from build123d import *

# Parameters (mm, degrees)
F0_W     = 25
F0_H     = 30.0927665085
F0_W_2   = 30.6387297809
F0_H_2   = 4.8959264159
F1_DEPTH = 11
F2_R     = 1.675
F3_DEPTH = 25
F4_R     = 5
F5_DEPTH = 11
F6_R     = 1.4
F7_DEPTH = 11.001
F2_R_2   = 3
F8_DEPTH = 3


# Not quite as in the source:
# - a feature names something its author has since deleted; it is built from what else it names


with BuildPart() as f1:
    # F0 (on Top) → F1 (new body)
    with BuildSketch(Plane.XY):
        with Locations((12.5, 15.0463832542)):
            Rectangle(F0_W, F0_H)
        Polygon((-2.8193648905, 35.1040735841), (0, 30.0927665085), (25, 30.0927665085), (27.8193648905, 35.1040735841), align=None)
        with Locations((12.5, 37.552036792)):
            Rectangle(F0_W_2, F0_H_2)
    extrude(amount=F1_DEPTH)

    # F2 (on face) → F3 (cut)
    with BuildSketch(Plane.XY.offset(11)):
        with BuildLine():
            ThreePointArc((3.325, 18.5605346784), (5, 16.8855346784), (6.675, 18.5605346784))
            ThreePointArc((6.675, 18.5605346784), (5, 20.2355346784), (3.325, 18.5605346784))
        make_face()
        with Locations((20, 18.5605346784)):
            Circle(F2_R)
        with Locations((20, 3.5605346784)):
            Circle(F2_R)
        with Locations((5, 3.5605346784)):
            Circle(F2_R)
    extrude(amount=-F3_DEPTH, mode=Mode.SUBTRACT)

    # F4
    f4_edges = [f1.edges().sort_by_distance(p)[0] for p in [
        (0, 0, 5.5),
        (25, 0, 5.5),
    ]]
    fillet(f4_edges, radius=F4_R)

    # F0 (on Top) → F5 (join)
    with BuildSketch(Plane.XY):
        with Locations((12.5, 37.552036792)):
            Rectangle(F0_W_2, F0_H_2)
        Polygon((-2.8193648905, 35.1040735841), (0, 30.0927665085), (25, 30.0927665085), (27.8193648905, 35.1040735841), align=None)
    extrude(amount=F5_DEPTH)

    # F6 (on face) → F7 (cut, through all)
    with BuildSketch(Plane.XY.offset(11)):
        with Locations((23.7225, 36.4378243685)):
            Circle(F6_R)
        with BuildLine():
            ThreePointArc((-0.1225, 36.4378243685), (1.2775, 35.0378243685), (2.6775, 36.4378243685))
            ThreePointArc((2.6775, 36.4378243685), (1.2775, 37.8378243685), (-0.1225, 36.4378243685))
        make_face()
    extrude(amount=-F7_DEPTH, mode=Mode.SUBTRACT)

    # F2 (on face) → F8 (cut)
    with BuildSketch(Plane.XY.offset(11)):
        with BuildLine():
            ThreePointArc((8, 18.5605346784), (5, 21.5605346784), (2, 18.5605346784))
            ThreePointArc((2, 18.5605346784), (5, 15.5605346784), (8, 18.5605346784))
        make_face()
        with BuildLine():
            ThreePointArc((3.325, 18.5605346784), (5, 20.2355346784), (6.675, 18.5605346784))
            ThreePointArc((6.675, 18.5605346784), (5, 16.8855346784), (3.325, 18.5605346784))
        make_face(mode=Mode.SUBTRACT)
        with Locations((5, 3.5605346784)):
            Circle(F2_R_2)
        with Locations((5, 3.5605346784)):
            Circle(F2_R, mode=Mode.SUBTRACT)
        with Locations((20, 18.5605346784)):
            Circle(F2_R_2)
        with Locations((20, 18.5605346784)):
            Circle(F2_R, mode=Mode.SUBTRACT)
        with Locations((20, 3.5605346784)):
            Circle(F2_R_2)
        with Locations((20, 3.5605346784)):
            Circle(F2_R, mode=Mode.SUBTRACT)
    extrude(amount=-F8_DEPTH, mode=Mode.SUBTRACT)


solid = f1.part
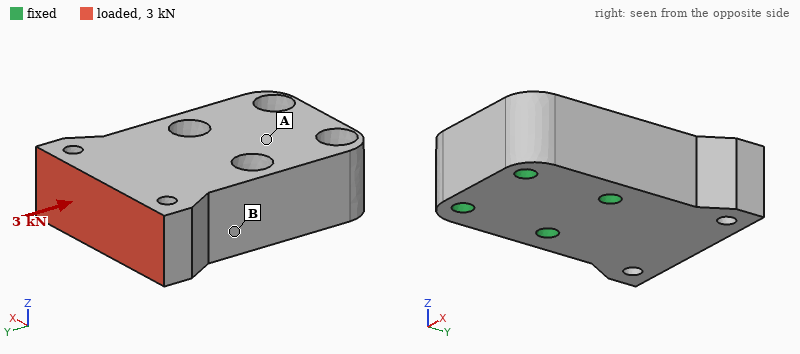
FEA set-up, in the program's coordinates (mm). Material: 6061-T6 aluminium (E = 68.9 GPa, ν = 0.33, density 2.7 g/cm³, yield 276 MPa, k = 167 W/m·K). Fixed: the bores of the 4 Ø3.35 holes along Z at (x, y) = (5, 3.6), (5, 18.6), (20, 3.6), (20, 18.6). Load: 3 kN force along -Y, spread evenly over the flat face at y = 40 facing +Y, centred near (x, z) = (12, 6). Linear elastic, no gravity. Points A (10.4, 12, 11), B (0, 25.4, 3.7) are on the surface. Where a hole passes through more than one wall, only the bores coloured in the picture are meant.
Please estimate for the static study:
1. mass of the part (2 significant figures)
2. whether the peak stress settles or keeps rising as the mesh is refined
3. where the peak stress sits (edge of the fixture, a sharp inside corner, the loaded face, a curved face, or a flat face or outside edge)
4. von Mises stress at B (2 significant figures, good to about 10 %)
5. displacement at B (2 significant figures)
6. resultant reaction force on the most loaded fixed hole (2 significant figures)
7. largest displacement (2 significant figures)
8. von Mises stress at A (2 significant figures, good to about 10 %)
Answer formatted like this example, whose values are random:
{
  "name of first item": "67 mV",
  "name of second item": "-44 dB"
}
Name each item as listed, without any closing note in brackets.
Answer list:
{
  "mass of the part": "29 g",
  "whether the peak stress settles or keeps rising as the mesh is refined": "keeps rising",
  "where the peak stress sits": "edge of the fixture",
  "von Mises stress at B": "13 MPa",
  "displacement at B": "1.6 µm",
  "resultant reaction force on the most loaded fixed hole": "1.3 kN",
  "largest displacement": "6.6 µm",
  "von Mises stress at A": "5.1 MPa"
}
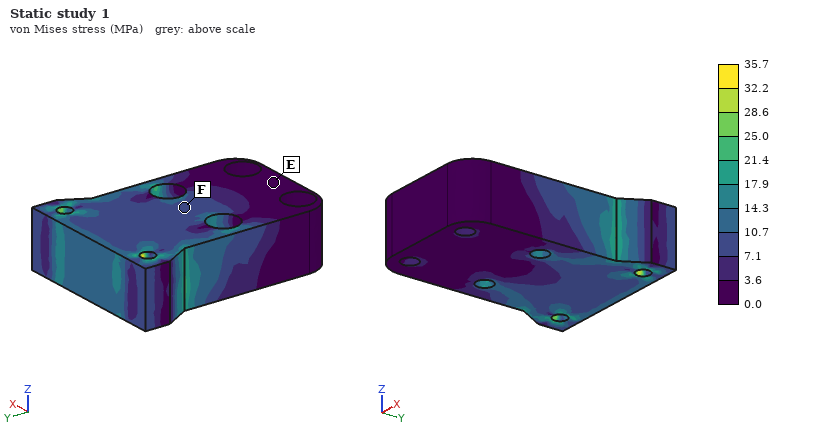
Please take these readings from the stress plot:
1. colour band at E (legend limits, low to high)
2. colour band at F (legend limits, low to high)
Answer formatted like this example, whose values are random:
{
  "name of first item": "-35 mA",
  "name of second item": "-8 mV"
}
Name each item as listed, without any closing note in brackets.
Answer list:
{
  "colour band at E": "0.0 to 3.6 MPa",
  "colour band at F": "7.1 to 10.7 MPa"
}
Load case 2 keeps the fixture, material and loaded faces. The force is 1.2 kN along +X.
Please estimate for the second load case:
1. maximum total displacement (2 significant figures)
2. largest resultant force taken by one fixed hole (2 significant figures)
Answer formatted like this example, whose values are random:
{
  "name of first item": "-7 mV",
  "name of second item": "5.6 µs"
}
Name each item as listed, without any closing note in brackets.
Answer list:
{
  "maximum total displacement": "12 µm",
  "largest resultant force taken by one fixed hole": "1.4 kN"
}
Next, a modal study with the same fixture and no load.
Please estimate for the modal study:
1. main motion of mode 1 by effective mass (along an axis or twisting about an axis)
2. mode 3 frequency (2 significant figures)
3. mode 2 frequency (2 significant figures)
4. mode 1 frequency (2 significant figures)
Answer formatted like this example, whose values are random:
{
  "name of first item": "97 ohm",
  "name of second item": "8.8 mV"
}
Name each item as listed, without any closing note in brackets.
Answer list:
{
  "main motion of mode 1 by effective mass": "along Z",
  "mode 3 frequency": "23 kHz",
  "mode 2 frequency": "22 kHz",
  "mode 1 frequency": "13 kHz"
}
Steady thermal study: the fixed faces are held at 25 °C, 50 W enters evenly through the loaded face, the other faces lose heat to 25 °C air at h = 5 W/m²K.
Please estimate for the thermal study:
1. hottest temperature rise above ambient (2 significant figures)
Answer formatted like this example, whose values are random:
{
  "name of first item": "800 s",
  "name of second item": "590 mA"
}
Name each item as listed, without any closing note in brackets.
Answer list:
{
  "hottest temperature rise above ambient": "25 K"
}
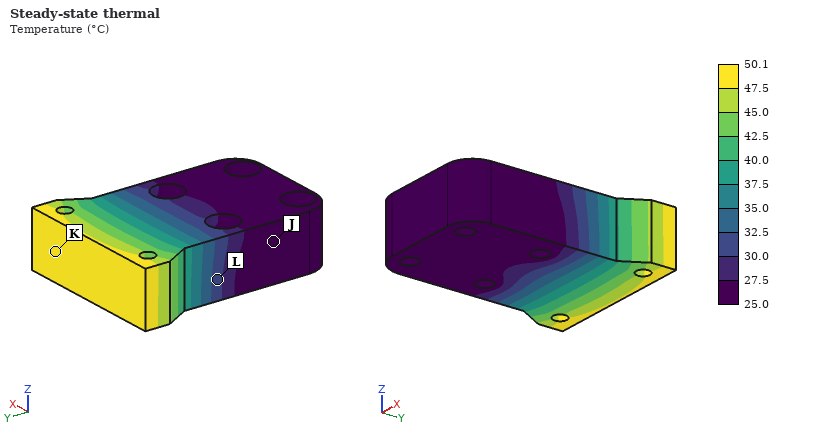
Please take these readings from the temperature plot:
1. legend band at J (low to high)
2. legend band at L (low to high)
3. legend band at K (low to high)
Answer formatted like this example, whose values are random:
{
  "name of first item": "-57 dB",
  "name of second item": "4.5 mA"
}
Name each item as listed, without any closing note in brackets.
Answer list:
{
  "legend band at J": "25.0 to 27.5 °C",
  "legend band at L": "30.0 to 32.5 °C",
  "legend band at K": "47.5 to 50.1 °C"
}
